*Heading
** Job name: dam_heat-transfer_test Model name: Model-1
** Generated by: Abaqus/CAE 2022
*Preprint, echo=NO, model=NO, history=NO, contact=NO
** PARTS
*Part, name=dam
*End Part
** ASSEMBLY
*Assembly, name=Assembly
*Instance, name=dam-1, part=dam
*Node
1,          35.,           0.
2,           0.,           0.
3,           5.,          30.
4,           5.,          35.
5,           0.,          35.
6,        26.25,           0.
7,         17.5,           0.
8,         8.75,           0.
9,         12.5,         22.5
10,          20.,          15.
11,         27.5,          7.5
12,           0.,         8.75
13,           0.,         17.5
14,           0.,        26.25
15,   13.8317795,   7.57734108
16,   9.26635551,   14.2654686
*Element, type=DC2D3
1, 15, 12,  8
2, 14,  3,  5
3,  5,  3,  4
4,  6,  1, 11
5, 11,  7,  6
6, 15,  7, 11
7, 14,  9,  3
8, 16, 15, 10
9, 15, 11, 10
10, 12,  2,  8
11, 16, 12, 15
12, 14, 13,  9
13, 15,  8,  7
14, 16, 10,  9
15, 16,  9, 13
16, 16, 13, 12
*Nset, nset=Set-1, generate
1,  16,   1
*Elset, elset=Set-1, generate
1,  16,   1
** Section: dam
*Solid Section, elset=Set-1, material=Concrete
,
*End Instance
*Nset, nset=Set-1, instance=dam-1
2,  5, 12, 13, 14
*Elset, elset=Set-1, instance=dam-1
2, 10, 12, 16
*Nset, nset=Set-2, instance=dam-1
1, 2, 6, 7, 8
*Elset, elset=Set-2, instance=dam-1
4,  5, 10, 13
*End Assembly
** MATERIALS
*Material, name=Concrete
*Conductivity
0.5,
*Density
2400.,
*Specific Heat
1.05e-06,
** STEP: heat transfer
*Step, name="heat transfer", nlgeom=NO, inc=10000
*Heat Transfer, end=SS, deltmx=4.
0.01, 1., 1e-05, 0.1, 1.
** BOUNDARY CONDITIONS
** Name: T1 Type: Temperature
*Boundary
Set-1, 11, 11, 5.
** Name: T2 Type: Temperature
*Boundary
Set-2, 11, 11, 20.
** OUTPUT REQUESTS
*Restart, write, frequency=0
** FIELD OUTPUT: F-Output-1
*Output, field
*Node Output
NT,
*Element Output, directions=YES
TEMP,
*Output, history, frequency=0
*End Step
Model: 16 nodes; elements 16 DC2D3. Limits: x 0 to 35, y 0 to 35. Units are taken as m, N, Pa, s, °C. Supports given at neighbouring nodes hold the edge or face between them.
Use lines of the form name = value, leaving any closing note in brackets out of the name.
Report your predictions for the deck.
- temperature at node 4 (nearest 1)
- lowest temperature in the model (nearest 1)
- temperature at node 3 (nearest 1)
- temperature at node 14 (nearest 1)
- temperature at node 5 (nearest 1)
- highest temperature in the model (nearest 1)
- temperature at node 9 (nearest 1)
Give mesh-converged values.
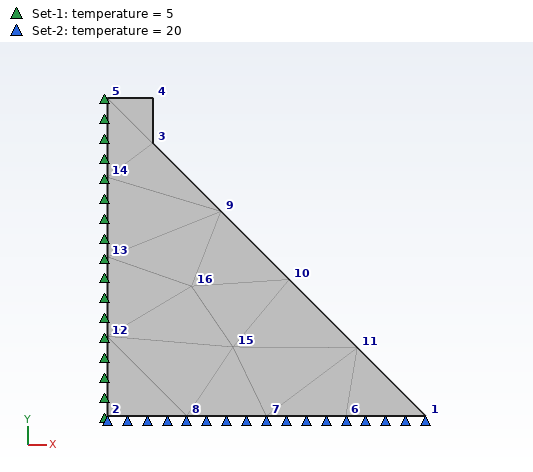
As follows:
temperature at node 4 = 5 °C
lowest temperature in the model = 5 °C
temperature at node 3 = 5 °C
temperature at node 14 = 5 °C
temperature at node 5 = 5 °C
highest temperature in the model = 20 °C
temperature at node 9 = 8 °C
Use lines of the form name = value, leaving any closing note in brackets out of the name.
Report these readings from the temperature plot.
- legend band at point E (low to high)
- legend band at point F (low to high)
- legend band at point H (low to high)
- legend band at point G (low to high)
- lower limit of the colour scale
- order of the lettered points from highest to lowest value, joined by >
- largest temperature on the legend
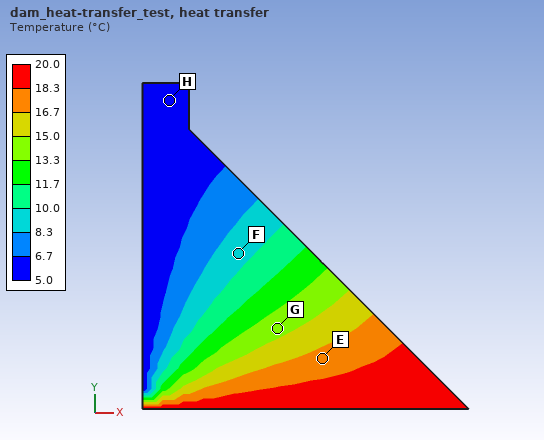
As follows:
legend band at point E = 16.7 to 18.3 °C
legend band at point F = 8.3 to 10.0 °C
legend band at point H = 5.0 to 6.7 °C
legend band at point G = 13.3 to 15.0 °C
lower limit of the colour scale = 5.0 °C
order of the lettered points from highest to lowest value, joined by > = E > G > F > H
largest temperature on the legend = 20.0 °C
